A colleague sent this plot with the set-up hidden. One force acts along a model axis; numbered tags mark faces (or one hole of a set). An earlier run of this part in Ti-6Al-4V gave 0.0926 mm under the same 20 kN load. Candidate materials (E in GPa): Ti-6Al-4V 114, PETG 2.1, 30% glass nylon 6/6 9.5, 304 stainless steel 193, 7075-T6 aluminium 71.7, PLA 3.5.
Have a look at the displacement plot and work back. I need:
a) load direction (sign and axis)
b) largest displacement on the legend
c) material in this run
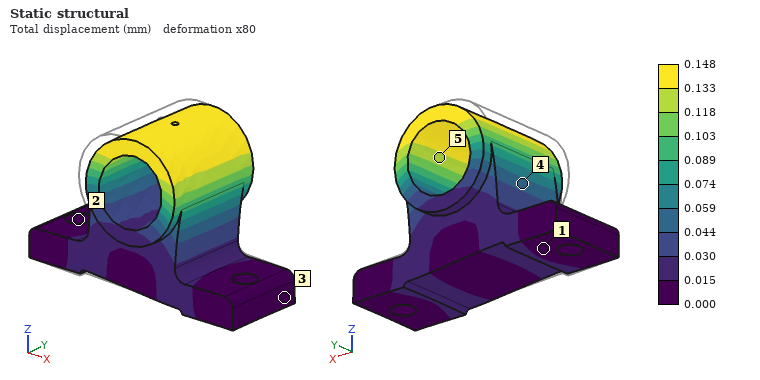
+X
0.148 mm
7075-T6 aluminium
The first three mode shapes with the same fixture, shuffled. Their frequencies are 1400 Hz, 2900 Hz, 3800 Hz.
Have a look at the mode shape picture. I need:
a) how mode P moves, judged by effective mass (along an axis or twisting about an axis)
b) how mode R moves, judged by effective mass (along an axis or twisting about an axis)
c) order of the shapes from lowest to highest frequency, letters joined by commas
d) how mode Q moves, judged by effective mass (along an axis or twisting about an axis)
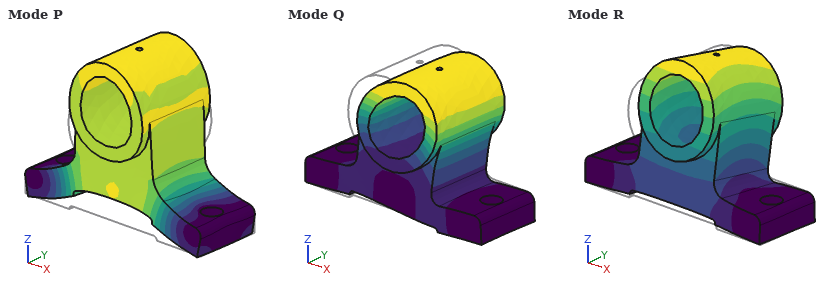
along Z
along Y
R, Q, P
along X
